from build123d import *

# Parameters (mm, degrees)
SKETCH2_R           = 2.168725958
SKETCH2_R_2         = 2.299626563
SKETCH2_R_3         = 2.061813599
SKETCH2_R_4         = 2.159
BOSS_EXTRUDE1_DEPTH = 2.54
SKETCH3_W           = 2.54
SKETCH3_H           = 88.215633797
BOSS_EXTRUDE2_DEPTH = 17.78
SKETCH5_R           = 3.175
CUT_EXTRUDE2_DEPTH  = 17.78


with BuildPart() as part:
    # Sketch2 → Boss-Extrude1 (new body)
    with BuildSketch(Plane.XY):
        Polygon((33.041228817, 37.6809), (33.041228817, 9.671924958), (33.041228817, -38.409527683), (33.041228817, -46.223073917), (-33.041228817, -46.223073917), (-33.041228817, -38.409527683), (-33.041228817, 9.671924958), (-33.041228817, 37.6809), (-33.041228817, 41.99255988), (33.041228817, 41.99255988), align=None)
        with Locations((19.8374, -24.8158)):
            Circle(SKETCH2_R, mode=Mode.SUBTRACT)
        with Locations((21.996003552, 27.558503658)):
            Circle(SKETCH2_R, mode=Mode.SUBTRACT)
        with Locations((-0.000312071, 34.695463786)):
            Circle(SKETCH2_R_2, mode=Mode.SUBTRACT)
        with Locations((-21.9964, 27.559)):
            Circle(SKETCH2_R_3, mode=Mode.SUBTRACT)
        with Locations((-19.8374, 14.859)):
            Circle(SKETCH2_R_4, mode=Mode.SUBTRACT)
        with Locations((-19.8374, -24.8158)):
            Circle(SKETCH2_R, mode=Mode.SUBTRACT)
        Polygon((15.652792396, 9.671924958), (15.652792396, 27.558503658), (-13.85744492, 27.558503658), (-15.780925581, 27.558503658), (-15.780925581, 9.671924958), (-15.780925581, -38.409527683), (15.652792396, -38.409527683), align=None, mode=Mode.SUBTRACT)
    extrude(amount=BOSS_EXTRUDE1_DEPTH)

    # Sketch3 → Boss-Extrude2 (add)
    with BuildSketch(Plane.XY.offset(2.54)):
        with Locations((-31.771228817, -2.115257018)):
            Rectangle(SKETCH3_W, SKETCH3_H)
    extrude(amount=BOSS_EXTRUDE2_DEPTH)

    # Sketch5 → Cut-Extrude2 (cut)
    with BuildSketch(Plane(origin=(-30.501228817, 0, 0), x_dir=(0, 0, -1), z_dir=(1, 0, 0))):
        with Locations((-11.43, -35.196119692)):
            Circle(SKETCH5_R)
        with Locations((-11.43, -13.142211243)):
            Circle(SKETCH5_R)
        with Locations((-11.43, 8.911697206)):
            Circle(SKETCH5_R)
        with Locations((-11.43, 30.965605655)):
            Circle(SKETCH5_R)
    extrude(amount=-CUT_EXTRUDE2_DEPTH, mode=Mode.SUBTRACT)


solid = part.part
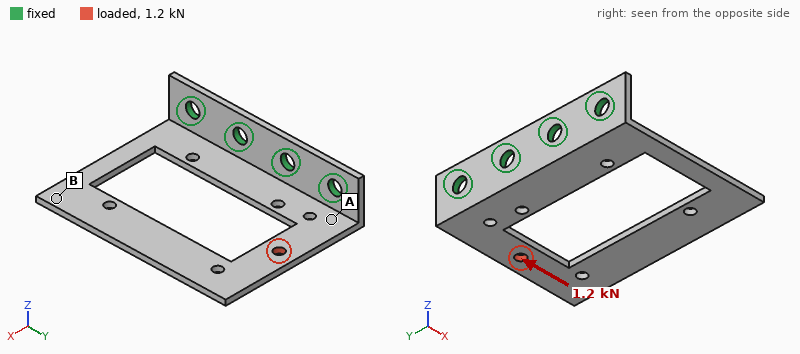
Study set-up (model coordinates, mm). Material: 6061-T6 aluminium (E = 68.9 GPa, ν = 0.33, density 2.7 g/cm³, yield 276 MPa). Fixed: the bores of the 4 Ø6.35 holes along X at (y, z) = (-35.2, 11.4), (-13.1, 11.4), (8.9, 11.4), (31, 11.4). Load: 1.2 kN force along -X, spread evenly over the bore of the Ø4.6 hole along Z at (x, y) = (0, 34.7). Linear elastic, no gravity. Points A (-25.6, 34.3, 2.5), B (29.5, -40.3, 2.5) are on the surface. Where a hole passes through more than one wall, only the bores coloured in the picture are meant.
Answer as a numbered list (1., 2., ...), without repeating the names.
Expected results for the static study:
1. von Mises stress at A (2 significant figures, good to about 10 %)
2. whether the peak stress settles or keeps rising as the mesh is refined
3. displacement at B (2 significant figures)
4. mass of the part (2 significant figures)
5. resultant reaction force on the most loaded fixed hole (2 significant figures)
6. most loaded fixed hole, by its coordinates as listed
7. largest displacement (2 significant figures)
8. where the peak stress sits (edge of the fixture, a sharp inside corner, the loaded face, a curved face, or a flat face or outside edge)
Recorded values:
1. 56 MPa
2. keeps rising
3. 0.22 mm
4. 35 g
5. 1.0 kN
6. (31, 11.4)
7. 0.70 mm
8. edge of the fixture
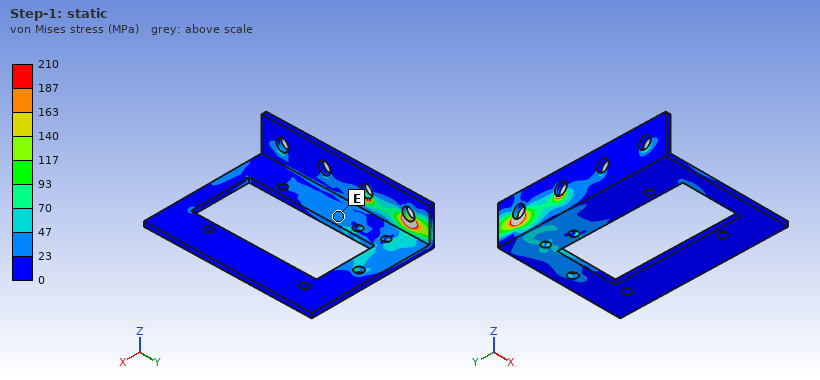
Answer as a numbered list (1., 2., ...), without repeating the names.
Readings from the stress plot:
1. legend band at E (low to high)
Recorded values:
1. 23 to 47 MPa
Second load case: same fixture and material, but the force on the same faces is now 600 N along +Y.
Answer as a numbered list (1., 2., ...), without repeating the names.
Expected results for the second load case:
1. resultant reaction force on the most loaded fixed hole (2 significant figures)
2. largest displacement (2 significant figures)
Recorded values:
1. 330 N
2. 0.22 mm
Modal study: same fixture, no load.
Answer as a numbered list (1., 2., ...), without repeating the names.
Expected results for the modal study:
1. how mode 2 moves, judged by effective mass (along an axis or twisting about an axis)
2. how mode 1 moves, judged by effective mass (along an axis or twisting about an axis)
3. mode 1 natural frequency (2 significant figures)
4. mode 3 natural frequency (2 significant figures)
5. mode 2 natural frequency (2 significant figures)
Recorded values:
1. twisting about X
2. along Z
3. 300 Hz
4. 1800 Hz
5. 700 Hz
